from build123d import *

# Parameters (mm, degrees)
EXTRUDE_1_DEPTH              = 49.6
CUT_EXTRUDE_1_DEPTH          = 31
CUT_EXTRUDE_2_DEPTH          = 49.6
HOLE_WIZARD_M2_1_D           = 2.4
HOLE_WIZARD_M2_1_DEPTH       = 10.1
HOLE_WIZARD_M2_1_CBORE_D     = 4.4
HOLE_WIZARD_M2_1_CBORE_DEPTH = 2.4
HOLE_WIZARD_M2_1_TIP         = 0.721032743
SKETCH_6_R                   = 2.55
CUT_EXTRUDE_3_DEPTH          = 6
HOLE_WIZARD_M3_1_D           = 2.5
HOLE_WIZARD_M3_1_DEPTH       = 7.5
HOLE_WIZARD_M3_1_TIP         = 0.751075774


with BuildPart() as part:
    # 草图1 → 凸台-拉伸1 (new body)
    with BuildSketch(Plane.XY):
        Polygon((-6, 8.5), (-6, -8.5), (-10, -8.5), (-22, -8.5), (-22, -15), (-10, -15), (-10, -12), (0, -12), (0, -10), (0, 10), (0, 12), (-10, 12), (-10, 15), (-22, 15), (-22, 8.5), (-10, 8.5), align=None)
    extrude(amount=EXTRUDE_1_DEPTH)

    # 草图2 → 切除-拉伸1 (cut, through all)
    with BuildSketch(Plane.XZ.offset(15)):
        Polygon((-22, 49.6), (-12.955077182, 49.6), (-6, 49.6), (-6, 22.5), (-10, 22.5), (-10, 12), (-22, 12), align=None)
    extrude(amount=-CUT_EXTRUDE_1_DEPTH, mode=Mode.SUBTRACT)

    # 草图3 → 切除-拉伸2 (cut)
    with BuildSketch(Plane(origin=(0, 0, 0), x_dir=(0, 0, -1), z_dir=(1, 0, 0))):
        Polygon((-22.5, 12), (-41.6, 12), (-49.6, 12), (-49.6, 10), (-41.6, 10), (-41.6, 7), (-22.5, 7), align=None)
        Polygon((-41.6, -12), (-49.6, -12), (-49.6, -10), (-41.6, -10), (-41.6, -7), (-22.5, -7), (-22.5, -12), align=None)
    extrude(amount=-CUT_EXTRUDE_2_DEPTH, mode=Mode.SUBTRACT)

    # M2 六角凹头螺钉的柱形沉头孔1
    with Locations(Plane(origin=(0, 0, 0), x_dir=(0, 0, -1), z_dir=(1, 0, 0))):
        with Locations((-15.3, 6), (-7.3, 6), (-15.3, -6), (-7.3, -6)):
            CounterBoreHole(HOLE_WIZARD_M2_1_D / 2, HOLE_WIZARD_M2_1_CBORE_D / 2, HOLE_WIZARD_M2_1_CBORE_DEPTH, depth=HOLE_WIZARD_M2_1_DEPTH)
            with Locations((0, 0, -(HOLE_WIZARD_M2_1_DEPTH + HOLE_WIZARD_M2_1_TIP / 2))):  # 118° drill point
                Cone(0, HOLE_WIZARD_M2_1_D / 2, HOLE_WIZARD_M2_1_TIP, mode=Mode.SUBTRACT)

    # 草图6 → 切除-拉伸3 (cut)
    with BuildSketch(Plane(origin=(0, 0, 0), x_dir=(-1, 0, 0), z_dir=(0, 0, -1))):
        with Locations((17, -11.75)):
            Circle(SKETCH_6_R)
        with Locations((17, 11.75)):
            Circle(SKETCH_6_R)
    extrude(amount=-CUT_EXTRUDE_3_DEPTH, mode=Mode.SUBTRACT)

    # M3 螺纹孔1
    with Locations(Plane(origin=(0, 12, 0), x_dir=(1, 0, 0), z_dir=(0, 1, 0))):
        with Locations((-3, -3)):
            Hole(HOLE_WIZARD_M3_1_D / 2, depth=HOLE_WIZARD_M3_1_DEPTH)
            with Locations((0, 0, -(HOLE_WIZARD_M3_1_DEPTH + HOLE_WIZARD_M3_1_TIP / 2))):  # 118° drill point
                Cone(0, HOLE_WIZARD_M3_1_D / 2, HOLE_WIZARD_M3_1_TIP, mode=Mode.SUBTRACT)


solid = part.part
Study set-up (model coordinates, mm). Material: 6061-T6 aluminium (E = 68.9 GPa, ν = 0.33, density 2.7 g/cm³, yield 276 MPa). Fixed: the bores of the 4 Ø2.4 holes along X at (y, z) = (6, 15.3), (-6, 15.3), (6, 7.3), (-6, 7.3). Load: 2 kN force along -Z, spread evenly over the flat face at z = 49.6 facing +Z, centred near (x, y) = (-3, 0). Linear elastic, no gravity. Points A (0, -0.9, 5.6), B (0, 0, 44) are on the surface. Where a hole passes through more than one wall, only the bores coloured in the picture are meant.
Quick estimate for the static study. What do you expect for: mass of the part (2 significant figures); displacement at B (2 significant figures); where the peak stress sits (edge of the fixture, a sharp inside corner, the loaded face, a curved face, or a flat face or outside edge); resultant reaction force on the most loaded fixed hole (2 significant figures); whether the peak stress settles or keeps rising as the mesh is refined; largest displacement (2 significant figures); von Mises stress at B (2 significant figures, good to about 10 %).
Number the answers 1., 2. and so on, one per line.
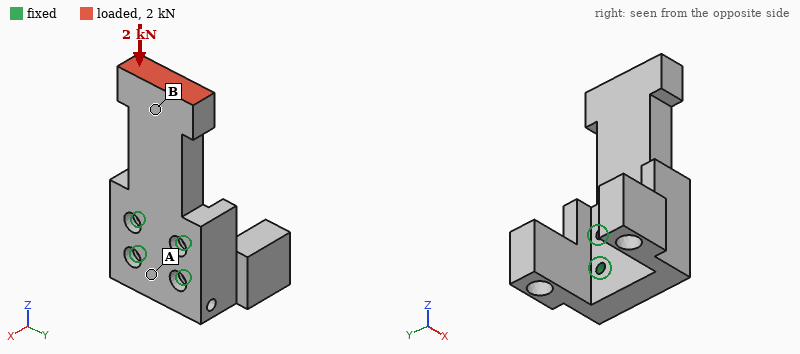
1. 21 g
2. 15 µm
3. edge of the fixture
4. 770 N
5. keeps rising
6. 19 µm
7. 18 MPa
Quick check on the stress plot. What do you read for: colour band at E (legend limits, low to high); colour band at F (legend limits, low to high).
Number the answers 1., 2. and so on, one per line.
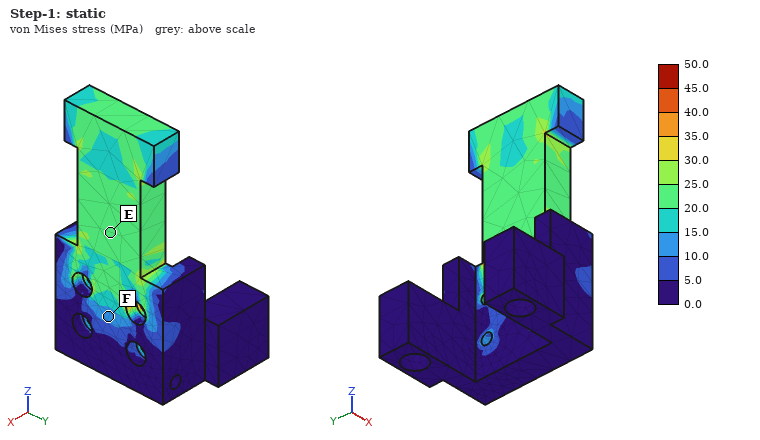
1. 20.0 to 25.0 MPa
2. 10.0 to 15.0 MPa
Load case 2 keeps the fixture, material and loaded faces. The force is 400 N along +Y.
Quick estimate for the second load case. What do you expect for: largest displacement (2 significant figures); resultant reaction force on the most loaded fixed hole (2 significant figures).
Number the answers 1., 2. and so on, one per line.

1. 57 µm
2. 790 N
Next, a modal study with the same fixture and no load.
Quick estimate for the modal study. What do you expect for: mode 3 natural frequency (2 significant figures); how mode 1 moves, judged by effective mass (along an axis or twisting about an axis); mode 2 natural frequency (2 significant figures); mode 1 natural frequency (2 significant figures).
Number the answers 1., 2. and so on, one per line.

1. 7000 Hz
2. along X
3. 6900 Hz
4. 3600 Hz
